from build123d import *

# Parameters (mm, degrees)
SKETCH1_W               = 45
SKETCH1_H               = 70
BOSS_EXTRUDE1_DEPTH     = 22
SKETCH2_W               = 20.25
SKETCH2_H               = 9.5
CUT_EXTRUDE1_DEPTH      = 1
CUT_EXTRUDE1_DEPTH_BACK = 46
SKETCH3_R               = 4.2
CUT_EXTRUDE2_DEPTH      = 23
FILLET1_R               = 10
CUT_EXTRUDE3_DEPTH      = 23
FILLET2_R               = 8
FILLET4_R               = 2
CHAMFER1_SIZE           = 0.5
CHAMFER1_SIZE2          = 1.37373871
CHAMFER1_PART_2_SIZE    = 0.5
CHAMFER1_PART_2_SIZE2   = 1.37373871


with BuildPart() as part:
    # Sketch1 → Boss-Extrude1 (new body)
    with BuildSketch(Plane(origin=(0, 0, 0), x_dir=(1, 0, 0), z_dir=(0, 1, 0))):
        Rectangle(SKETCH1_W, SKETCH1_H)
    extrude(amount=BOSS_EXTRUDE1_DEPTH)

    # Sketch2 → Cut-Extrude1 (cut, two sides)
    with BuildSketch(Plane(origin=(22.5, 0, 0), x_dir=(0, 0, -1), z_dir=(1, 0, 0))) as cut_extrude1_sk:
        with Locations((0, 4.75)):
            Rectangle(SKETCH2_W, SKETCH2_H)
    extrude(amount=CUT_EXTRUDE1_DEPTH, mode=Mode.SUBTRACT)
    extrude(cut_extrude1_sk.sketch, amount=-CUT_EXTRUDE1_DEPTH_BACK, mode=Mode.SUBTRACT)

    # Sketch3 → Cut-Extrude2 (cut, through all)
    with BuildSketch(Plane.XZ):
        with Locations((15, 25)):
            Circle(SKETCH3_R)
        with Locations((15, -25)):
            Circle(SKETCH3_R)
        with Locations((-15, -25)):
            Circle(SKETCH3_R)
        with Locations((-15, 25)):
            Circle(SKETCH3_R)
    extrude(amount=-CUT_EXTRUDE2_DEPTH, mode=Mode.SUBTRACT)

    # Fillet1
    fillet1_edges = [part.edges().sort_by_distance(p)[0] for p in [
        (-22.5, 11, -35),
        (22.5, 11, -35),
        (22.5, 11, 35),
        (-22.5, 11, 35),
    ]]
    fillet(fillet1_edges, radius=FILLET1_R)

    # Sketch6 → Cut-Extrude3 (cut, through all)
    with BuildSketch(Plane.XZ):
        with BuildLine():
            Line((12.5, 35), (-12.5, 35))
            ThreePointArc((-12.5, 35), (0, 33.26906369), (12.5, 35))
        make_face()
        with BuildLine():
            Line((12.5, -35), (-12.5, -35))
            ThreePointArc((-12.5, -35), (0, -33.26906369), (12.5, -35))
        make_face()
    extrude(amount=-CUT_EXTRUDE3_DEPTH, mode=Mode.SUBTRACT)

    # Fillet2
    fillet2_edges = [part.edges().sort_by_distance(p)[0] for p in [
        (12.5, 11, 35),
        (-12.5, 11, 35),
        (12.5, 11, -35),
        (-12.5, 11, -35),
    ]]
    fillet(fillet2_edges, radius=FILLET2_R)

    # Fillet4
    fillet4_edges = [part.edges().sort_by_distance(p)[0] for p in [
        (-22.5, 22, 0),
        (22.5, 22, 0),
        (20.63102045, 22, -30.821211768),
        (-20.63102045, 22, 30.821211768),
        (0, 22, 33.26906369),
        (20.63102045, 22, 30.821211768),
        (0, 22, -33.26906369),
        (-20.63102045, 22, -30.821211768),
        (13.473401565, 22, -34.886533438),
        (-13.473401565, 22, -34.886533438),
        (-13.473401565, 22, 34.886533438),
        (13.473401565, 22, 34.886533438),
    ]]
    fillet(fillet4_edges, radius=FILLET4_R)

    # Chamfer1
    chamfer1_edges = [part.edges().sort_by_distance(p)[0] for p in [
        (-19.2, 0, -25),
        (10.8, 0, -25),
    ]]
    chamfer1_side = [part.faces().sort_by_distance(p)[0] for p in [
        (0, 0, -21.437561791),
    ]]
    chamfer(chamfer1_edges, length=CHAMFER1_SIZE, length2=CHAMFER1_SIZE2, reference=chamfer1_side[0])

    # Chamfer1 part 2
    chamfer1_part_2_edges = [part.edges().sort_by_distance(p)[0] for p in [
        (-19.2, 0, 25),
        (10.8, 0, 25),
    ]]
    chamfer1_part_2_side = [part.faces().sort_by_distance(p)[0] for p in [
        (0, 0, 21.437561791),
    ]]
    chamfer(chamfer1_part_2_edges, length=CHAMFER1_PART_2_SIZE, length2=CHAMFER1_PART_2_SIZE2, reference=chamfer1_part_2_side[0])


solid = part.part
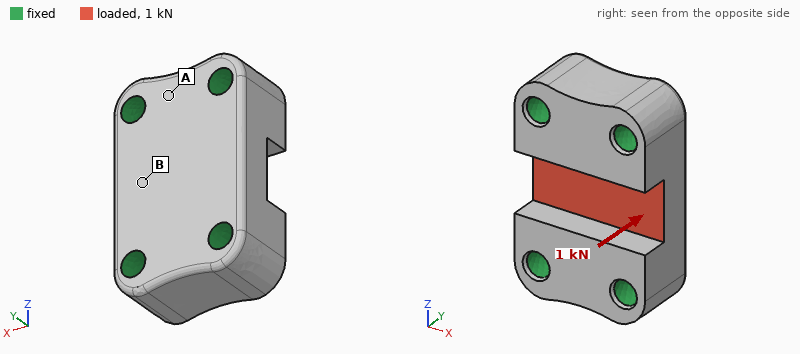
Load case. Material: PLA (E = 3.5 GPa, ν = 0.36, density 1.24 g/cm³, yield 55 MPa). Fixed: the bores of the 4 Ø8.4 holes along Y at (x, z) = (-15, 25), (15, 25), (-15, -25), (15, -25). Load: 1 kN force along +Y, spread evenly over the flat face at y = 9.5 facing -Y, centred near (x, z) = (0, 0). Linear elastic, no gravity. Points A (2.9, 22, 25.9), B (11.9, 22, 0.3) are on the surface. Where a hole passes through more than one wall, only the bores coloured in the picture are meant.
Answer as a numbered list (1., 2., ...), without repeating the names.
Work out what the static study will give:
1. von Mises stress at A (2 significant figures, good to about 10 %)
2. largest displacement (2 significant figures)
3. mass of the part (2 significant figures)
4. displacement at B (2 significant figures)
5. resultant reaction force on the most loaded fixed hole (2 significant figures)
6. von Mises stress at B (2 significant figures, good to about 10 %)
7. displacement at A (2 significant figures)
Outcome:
1. 0.49 MPa
2. 20 µm
3. 65 g
4. 16 µm
5. 260 N
6. 2.1 MPa
7. 3.1 µm
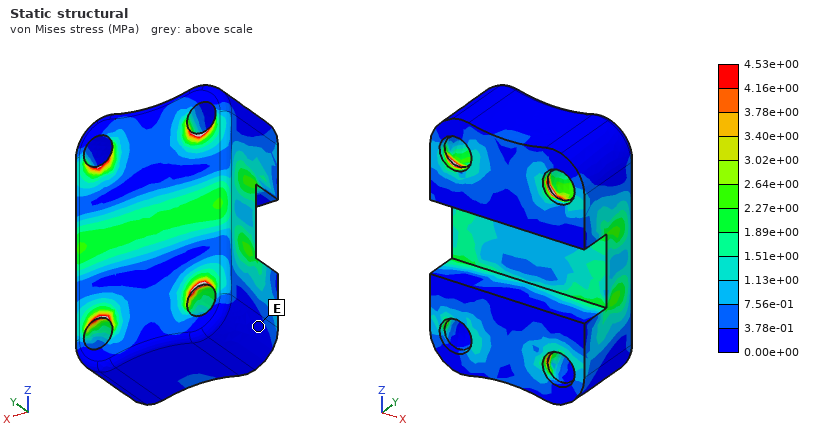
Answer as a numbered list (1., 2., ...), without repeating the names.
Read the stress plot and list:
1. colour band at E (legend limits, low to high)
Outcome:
1. 0.00e+00 to 3.78e-01 MPa
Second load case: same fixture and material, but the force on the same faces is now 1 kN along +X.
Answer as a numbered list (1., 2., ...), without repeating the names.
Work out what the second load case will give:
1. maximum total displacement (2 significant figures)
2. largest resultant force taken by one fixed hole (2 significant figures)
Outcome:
1. 24 µm
2. 290 N
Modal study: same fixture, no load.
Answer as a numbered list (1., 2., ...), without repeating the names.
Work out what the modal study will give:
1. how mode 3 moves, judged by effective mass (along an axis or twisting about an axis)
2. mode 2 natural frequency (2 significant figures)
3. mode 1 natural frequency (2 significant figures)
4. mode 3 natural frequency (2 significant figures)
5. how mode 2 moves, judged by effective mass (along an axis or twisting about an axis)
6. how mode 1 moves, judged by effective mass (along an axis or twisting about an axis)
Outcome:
1. along X
2. 11 kHz
3. 9100 Hz
4. 12 kHz
5. along X
6. along Y
